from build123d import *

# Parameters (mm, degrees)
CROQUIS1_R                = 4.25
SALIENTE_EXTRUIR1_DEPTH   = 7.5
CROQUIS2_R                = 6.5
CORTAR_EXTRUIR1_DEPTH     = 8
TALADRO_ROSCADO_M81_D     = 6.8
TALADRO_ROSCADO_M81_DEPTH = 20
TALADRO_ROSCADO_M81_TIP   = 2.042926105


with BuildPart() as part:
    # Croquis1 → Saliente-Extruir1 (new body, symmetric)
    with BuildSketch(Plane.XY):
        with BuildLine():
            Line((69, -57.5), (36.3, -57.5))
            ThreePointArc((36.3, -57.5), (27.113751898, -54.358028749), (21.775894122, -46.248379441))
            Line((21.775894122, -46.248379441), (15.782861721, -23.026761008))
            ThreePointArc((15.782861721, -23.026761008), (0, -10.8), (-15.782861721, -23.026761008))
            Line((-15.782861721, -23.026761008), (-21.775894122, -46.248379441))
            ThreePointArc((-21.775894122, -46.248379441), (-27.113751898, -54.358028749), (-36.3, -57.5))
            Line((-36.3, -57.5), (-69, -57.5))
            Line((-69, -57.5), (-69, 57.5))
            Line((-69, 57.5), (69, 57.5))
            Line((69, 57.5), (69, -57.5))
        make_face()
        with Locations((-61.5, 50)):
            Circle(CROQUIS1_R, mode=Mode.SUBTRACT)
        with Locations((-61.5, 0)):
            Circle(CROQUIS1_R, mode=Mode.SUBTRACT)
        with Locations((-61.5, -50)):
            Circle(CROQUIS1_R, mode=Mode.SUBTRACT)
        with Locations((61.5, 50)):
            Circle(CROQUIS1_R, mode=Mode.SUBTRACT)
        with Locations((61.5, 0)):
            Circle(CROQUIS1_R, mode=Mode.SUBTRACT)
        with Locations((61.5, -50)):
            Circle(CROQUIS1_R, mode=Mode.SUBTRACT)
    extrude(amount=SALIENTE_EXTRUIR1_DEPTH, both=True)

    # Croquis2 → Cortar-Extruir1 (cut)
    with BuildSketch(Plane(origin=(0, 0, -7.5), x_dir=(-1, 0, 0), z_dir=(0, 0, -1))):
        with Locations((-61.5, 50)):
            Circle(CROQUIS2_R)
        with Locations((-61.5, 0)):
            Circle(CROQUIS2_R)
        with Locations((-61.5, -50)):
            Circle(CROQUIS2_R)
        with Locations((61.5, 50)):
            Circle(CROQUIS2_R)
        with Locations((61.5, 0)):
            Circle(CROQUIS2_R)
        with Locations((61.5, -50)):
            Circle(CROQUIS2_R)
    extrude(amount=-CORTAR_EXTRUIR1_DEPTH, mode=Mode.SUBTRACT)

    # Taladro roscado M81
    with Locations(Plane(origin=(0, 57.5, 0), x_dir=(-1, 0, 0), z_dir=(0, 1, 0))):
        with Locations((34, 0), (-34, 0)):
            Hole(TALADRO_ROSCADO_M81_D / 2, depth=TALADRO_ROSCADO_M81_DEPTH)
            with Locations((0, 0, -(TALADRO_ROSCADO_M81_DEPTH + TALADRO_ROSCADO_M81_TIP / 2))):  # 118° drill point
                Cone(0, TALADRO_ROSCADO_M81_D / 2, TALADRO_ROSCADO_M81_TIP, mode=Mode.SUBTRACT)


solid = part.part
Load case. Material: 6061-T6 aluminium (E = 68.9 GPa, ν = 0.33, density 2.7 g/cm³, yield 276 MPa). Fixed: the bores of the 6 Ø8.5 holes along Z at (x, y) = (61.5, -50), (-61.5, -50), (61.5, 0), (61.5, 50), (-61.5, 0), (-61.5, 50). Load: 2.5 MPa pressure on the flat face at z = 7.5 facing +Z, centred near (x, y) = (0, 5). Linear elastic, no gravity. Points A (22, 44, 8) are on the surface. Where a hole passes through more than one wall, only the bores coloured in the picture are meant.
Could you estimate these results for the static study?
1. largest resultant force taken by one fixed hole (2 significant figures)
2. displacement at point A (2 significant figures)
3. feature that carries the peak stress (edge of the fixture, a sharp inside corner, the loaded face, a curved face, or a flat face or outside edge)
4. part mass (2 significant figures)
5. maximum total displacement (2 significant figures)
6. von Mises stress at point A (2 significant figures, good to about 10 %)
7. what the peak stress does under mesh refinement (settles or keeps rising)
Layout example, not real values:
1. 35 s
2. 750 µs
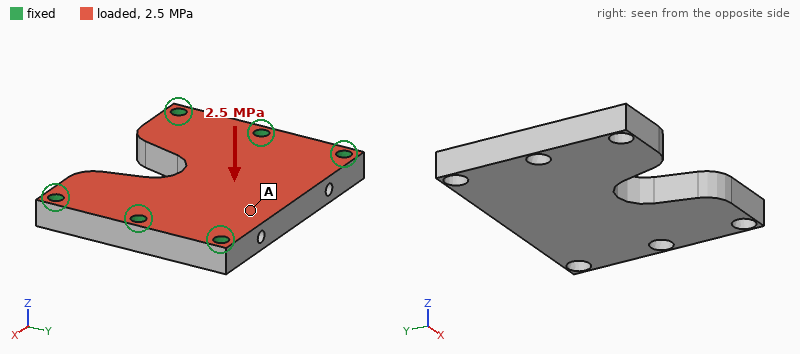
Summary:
1. 9.6 kN
2. 0.14 mm
3. edge of the fixture
4. 540 g
5. 0.18 mm
6. 35 MPa
7. keeps rising
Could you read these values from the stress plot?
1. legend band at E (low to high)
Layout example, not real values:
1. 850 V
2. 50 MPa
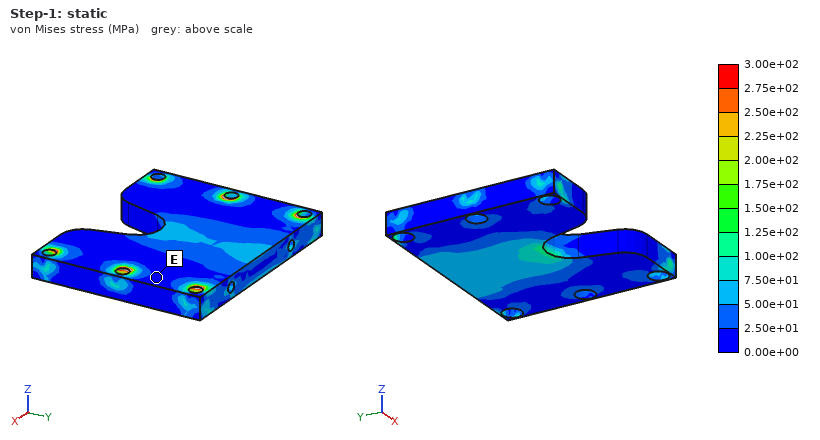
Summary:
1. 0.00e+00 to 2.50e+01 MPa
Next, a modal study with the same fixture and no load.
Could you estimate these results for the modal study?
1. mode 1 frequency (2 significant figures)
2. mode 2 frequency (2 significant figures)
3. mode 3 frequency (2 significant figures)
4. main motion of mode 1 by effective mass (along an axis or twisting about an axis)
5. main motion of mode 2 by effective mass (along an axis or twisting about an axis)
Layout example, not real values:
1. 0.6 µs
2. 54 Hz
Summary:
1. 3500 Hz
2. 5400 Hz
3. 7000 Hz
4. along Z
5. twisting about X
